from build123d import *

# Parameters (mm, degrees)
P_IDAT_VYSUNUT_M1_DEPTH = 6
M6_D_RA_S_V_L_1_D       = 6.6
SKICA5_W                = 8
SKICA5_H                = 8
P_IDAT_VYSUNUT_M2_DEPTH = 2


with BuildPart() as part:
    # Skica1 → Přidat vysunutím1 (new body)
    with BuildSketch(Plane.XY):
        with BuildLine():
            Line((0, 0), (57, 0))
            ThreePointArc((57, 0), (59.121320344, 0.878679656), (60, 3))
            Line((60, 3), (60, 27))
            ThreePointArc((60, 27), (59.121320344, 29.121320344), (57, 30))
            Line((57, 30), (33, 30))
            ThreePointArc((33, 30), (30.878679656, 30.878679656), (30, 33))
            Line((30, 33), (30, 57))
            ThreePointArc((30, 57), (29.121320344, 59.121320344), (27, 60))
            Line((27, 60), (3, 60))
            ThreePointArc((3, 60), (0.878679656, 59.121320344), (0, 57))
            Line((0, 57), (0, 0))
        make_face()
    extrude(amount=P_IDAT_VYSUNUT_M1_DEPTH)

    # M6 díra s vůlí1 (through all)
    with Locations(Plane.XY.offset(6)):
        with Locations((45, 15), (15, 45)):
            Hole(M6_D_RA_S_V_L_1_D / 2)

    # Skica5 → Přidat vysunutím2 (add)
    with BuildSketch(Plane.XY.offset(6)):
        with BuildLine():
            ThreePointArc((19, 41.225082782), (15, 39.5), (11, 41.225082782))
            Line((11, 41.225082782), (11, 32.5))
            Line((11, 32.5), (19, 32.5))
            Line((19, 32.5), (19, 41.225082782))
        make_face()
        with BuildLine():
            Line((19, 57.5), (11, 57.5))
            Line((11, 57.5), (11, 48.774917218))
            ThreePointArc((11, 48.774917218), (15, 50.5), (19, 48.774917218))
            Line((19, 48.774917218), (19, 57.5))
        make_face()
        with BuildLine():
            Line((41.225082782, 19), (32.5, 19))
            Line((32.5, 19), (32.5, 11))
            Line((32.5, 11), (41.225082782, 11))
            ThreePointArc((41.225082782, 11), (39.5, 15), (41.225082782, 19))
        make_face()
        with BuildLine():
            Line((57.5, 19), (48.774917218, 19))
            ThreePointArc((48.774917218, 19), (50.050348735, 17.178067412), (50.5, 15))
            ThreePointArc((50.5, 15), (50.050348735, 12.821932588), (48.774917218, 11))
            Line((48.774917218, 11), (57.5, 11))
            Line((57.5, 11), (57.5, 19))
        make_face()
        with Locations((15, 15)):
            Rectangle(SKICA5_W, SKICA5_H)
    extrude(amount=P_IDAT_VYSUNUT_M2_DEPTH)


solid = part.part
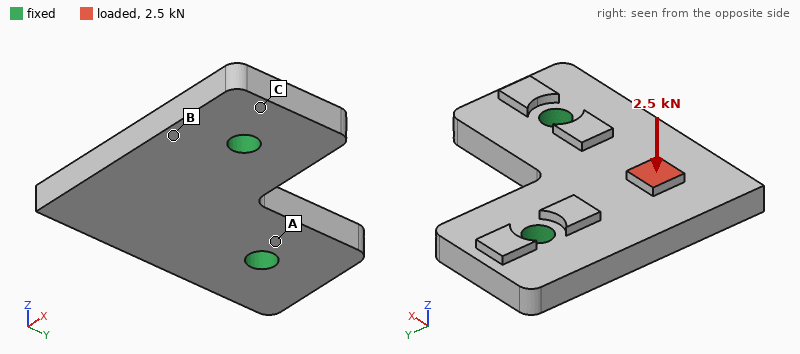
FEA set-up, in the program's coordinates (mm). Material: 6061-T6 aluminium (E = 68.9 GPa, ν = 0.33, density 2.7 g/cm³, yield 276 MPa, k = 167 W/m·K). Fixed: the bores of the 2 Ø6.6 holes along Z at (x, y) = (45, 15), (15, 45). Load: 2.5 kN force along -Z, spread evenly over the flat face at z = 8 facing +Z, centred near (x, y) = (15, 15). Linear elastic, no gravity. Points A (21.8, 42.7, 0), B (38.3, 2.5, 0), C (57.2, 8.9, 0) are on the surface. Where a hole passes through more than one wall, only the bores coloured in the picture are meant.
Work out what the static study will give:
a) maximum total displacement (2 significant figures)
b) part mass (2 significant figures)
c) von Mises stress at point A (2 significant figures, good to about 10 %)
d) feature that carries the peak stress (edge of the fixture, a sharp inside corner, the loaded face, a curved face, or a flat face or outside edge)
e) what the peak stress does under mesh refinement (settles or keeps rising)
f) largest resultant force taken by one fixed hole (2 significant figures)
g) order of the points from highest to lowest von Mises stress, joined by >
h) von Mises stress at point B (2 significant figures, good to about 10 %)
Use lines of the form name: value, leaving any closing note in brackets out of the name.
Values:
maximum total displacement: 0.37 mm
part mass: 44 g
von Mises stress at point A: 59 MPa
feature that carries the peak stress: edge of the fixture
what the peak stress does under mesh refinement: keeps rising
largest resultant force taken by one fixed hole: 1.3 kN
order of the points from highest to lowest von Mises stress, joined by >: B > A > C
von Mises stress at point B: 92 MPa
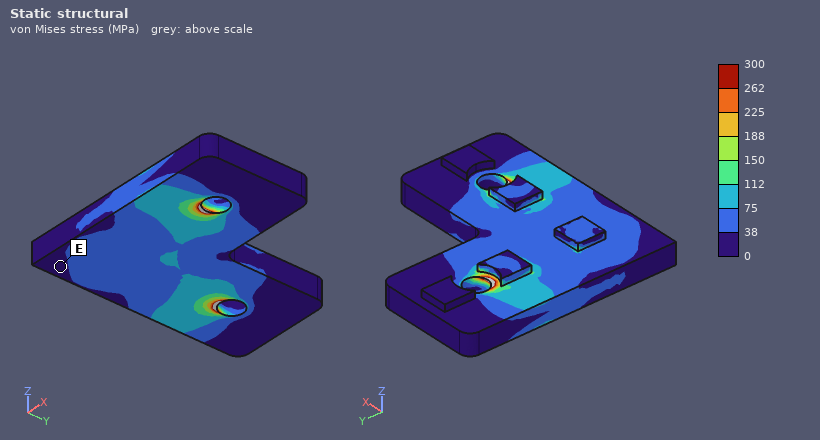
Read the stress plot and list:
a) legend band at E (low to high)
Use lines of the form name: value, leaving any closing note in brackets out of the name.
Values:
legend band at E: 0 to 38 MPa
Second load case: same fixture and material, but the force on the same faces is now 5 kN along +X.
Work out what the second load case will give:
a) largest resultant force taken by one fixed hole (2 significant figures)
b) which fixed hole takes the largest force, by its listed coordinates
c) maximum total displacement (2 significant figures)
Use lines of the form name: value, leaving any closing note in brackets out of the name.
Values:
largest resultant force taken by one fixed hole: 4.4 kN
which fixed hole takes the largest force, by its listed coordinates: (45, 15)
maximum total displacement: 0.20 mm
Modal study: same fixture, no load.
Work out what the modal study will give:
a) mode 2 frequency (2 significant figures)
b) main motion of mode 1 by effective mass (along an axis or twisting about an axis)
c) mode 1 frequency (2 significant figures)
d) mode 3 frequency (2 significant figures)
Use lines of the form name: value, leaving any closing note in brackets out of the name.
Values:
mode 2 frequency: 14 kHz
main motion of mode 1 by effective mass: along Z
mode 1 frequency: 4500 Hz
mode 3 frequency: 16 kHz
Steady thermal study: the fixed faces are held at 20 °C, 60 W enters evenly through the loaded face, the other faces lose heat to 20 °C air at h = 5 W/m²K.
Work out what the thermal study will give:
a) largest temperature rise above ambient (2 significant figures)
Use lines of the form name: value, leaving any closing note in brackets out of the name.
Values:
largest temperature rise above ambient: 57 K
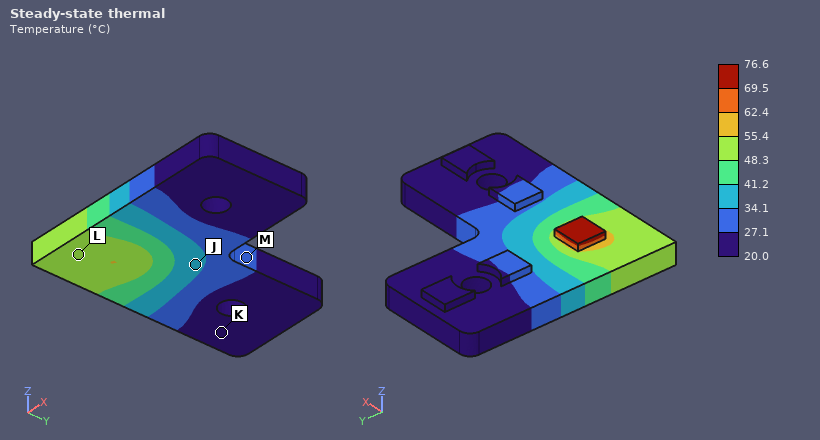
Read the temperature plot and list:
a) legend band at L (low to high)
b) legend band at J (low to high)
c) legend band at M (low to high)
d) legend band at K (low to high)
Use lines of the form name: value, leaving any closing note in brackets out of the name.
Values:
legend band at L: 48.3 to 55.4 °C
legend band at J: 34.1 to 41.2 °C
legend band at M: 27.1 to 34.1 °C
legend band at K: 20.0 to 27.1 °C
